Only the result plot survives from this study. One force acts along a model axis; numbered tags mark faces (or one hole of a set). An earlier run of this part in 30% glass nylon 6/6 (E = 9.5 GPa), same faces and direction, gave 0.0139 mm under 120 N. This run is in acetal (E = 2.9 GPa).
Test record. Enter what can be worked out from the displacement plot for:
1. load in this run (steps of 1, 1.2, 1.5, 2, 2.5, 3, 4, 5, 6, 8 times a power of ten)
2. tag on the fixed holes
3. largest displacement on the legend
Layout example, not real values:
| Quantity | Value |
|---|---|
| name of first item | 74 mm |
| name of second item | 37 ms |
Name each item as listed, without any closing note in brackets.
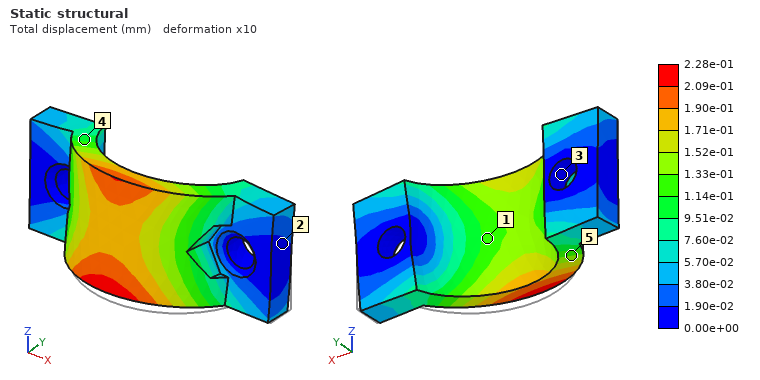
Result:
| Quantity | Value |
|---|---|
| load in this run | 600 N |
| tag on the fixed holes | 3 |
| largest displacement on the legend | 2.28e-01 mm |
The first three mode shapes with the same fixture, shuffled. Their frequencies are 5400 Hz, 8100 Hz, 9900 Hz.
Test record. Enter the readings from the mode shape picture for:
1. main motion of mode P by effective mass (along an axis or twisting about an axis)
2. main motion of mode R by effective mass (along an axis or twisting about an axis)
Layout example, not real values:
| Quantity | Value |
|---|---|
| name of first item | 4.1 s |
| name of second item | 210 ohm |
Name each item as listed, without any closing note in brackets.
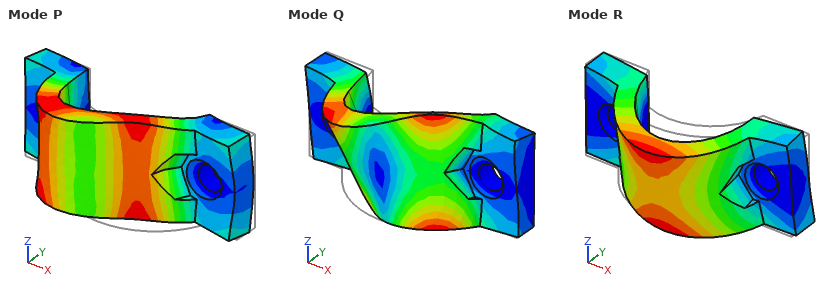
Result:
| Quantity | Value |
|---|---|
| main motion of mode P by effective mass | along X |
| main motion of mode R by effective mass | along Z |
